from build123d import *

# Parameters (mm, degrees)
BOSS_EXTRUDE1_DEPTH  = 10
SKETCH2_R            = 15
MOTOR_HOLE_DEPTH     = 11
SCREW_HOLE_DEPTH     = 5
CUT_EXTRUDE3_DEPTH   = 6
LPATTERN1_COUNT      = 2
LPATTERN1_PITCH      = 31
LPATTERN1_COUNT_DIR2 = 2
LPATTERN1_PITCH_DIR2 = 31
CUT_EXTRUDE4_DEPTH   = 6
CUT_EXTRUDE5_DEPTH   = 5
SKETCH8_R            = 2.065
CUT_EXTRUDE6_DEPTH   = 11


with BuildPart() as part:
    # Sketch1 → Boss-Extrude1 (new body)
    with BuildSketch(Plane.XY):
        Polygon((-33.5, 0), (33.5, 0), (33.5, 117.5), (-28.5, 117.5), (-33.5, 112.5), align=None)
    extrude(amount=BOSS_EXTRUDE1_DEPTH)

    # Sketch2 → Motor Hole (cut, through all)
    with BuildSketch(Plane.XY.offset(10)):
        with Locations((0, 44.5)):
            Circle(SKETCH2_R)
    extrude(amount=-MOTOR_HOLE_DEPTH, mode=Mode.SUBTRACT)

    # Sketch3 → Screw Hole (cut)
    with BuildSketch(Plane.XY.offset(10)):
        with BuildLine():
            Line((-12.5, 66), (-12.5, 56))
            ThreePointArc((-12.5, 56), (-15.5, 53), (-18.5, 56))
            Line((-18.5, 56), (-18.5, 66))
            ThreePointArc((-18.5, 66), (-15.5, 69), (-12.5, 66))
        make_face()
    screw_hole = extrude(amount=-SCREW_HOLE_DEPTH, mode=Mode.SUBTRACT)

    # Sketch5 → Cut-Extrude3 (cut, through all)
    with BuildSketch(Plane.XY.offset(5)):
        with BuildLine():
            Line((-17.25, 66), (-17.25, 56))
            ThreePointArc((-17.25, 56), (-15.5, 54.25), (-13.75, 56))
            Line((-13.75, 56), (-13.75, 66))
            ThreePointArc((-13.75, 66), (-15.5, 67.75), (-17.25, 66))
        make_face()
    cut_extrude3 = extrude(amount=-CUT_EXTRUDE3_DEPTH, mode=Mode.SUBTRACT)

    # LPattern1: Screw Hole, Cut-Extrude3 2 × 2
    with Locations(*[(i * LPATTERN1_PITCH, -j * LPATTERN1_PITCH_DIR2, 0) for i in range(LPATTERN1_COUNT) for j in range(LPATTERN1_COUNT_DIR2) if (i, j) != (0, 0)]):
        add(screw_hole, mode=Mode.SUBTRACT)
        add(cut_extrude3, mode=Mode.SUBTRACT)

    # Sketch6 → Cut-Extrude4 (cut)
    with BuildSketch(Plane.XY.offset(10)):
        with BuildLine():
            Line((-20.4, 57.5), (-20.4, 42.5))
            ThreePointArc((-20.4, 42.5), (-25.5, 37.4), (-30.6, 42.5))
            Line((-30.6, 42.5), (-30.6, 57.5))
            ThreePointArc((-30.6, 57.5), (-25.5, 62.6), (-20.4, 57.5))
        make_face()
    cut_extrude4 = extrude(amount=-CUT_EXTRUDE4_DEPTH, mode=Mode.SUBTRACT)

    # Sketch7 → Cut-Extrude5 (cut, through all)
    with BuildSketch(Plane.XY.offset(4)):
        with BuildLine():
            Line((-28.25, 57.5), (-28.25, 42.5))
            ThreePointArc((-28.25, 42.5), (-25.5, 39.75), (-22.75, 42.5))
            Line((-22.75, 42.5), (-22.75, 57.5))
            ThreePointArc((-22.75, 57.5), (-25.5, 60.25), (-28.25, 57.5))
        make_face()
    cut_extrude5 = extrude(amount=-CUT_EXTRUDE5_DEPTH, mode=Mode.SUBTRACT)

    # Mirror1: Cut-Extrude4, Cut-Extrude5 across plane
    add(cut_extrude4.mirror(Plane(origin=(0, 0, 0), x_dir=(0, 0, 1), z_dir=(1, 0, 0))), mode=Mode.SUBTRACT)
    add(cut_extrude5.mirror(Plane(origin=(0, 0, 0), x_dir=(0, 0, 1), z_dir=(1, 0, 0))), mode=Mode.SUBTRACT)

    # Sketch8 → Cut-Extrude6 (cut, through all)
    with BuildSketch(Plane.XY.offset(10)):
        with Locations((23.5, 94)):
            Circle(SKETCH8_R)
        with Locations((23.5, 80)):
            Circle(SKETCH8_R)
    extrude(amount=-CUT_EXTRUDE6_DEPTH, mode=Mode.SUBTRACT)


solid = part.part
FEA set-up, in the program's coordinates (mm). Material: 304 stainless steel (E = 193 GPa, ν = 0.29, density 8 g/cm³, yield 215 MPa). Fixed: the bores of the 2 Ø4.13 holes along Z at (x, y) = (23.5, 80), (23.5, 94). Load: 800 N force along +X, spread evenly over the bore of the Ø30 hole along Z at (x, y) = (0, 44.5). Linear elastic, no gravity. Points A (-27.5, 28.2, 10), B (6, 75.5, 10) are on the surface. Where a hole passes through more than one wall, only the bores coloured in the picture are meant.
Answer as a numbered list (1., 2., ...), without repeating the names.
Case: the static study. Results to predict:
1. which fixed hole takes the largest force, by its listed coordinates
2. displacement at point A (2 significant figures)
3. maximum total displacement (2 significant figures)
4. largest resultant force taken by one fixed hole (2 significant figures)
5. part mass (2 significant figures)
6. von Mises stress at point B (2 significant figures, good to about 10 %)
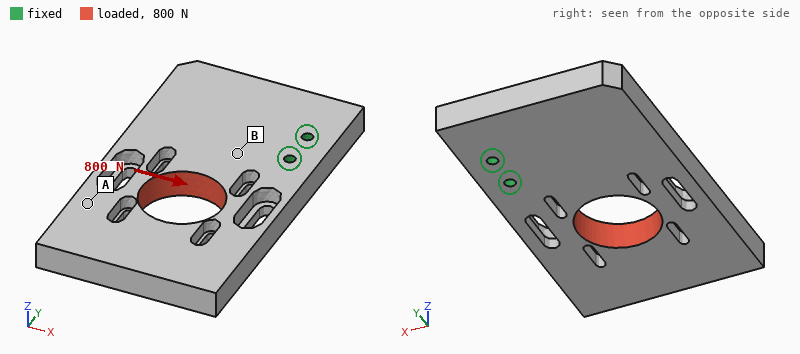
1. (23.5, 80)
2. 13 µm
3. 17 µm
4. 2.3 kN
5. 520 g
6. 6.6 MPa
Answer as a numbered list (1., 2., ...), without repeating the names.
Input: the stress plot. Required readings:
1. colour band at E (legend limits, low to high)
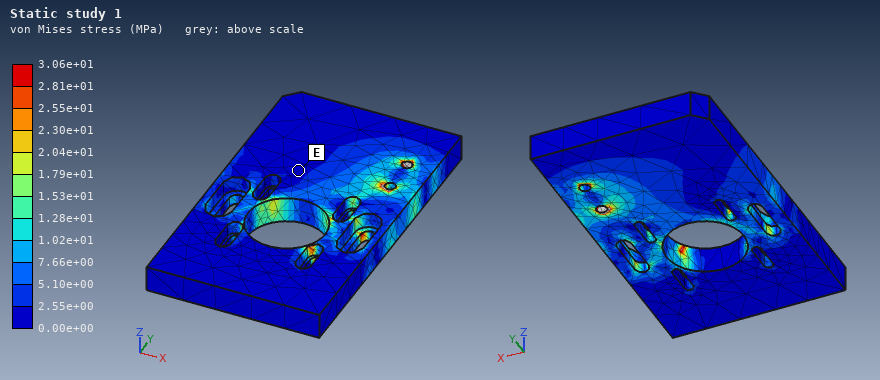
1. 0.00e+00 to 2.55e+00 MPa
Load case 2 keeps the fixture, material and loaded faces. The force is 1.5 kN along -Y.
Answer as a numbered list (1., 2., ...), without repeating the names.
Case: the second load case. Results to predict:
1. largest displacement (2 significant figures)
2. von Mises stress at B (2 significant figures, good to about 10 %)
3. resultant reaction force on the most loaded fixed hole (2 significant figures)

1. 15 µm
2. 6.7 MPa
3. 2.2 kN
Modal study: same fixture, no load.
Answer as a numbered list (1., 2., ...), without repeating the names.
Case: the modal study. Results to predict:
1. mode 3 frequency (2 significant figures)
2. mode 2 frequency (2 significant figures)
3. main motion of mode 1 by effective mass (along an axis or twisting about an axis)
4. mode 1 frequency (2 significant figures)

1. 1900 Hz
2. 1600 Hz
3. along Z
4. 760 Hz
